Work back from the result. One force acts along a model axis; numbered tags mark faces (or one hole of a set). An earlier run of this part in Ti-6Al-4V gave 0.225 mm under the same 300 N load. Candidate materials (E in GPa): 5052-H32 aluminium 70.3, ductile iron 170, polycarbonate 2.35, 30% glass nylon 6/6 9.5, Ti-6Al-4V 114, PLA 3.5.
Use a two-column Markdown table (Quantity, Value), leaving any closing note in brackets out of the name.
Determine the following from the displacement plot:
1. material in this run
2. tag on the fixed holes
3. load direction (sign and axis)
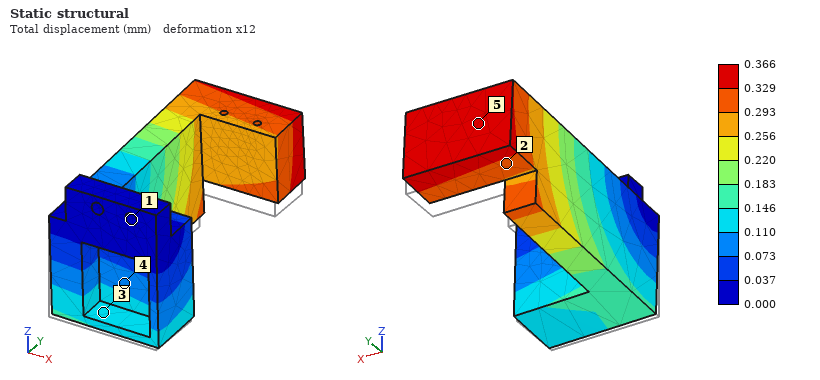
| Quantity | Value |
|---|---|
| material in this run | 5052-H32 aluminium |
| tag on the fixed holes | 1 |
| load direction | +Z |
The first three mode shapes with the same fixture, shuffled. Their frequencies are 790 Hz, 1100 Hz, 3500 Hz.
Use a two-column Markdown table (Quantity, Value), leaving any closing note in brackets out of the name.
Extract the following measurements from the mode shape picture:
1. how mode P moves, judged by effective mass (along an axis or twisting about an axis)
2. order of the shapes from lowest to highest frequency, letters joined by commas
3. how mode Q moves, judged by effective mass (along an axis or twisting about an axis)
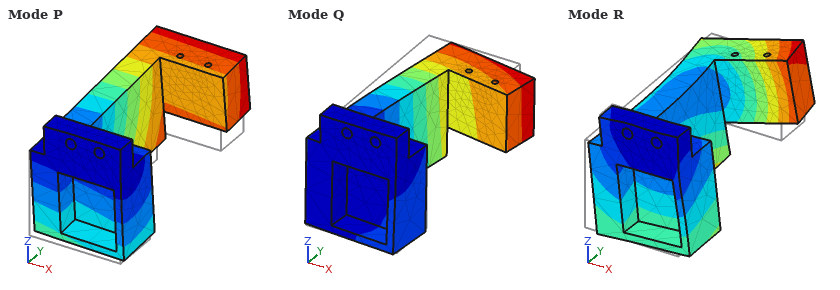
| Quantity | Value |
|---|---|
| how mode P moves, judged by effective mass | along Z |
| order of the shapes from lowest to highest frequency, letters joined by commas | P, Q, R |
| how mode Q moves, judged by effective mass | along X |
